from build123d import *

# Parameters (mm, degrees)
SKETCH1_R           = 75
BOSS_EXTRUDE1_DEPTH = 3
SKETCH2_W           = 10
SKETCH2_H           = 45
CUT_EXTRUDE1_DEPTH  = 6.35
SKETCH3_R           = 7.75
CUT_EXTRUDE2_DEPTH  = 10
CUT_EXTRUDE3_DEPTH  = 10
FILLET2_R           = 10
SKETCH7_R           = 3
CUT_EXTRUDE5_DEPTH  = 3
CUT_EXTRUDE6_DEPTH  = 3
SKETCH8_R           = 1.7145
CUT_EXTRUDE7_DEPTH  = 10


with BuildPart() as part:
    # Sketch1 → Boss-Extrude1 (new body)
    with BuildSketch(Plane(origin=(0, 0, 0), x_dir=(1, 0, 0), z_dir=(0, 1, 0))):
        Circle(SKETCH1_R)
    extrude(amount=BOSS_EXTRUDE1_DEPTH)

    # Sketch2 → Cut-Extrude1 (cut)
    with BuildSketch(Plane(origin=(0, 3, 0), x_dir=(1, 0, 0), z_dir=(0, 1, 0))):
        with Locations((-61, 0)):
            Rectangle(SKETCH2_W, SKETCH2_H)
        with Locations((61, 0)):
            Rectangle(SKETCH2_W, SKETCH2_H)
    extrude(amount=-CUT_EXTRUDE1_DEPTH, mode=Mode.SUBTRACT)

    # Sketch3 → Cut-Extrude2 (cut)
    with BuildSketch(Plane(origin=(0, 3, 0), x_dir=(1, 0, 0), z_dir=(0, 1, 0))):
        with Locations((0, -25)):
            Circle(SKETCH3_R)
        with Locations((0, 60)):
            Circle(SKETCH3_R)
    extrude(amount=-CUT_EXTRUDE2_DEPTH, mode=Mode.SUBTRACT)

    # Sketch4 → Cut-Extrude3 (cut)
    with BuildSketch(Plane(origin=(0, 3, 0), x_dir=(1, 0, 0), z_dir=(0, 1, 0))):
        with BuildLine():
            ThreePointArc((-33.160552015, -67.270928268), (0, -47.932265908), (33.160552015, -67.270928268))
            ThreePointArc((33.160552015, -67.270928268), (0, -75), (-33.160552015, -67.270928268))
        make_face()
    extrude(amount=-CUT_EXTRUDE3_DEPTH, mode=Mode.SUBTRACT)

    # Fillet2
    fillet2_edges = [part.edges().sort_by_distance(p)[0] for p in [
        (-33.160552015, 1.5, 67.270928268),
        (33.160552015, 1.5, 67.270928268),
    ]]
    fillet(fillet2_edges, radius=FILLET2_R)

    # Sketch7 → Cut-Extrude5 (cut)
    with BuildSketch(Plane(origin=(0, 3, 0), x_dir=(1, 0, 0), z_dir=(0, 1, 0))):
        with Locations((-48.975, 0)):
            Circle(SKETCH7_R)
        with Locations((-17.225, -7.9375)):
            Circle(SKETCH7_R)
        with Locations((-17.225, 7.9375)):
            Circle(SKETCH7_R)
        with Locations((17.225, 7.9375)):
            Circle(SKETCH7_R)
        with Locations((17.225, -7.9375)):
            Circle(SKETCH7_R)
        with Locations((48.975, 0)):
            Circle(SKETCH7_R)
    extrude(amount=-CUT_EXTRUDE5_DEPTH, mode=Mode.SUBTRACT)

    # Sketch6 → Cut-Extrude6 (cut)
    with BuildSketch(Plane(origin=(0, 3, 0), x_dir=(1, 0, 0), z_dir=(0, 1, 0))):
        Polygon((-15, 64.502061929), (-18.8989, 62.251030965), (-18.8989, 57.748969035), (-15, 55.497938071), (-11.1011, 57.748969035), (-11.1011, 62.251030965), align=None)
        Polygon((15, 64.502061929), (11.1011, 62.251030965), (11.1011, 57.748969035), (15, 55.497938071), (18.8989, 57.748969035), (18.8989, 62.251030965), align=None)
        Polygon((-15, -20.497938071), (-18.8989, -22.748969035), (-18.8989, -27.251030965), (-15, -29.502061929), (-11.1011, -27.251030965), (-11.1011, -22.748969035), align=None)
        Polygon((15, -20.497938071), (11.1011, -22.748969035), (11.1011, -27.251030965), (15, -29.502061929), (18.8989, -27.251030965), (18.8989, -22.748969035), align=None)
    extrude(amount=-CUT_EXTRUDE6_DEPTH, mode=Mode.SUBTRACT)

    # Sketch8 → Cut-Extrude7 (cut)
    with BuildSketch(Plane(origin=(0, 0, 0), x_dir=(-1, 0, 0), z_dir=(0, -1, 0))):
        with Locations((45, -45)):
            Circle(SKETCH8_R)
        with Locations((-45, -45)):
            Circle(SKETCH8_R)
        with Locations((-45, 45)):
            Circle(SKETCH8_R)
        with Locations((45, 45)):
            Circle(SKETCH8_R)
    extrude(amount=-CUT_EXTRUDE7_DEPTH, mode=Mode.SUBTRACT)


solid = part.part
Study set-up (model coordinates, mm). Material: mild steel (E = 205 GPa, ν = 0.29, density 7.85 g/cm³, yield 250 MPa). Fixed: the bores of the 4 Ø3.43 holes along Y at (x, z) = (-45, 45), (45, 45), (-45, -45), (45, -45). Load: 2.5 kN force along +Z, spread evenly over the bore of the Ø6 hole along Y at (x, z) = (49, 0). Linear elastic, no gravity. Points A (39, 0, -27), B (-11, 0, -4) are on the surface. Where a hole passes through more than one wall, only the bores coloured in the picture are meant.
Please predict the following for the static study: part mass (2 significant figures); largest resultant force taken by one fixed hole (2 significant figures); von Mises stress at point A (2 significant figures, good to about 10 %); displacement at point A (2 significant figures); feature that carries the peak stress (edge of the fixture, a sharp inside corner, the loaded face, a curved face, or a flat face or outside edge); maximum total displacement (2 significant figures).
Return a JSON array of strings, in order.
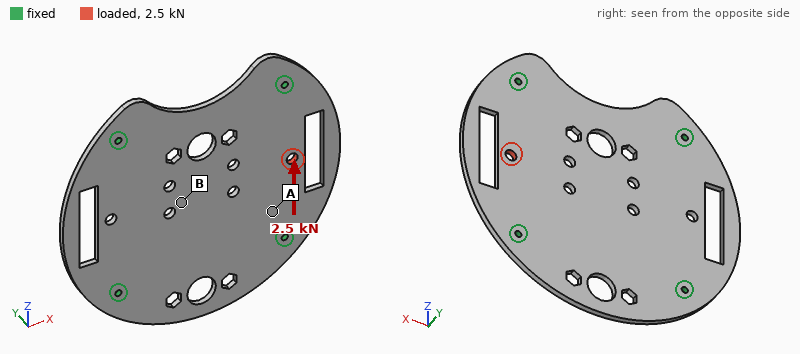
["350 g", "1.2 kN", "12 MPa", "1.8 µm", "the loaded face", "5.4 µm"]
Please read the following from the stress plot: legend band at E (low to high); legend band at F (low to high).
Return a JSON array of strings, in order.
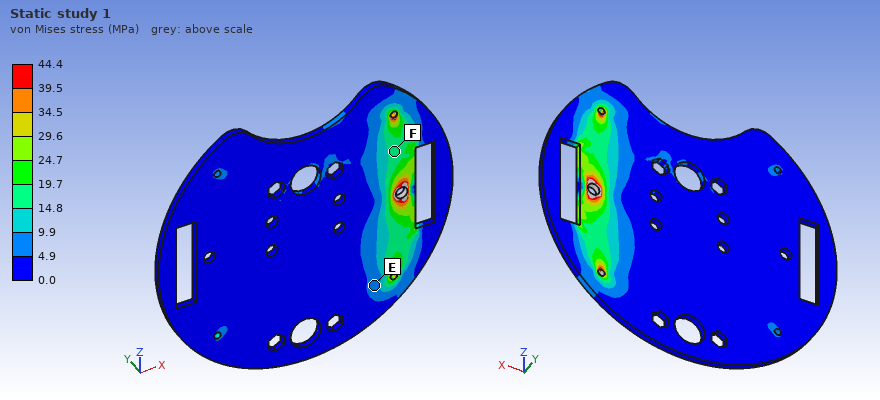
["4.9 to 9.9 MPa", "14.8 to 19.7 MPa"]
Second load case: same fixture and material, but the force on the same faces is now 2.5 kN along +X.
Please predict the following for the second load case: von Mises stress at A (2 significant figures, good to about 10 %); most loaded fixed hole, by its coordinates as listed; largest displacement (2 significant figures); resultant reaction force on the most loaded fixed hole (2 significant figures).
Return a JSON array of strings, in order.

["9.2 MPa", "(45, -45)", "9.5 µm", "800 N"]
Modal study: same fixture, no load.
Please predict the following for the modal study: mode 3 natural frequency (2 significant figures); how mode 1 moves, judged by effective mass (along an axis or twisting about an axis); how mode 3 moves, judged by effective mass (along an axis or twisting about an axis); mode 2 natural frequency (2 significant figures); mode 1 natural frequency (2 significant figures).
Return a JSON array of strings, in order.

["1700 Hz", "along Y", "twisting about Z", "1500 Hz", "1300 Hz"]
